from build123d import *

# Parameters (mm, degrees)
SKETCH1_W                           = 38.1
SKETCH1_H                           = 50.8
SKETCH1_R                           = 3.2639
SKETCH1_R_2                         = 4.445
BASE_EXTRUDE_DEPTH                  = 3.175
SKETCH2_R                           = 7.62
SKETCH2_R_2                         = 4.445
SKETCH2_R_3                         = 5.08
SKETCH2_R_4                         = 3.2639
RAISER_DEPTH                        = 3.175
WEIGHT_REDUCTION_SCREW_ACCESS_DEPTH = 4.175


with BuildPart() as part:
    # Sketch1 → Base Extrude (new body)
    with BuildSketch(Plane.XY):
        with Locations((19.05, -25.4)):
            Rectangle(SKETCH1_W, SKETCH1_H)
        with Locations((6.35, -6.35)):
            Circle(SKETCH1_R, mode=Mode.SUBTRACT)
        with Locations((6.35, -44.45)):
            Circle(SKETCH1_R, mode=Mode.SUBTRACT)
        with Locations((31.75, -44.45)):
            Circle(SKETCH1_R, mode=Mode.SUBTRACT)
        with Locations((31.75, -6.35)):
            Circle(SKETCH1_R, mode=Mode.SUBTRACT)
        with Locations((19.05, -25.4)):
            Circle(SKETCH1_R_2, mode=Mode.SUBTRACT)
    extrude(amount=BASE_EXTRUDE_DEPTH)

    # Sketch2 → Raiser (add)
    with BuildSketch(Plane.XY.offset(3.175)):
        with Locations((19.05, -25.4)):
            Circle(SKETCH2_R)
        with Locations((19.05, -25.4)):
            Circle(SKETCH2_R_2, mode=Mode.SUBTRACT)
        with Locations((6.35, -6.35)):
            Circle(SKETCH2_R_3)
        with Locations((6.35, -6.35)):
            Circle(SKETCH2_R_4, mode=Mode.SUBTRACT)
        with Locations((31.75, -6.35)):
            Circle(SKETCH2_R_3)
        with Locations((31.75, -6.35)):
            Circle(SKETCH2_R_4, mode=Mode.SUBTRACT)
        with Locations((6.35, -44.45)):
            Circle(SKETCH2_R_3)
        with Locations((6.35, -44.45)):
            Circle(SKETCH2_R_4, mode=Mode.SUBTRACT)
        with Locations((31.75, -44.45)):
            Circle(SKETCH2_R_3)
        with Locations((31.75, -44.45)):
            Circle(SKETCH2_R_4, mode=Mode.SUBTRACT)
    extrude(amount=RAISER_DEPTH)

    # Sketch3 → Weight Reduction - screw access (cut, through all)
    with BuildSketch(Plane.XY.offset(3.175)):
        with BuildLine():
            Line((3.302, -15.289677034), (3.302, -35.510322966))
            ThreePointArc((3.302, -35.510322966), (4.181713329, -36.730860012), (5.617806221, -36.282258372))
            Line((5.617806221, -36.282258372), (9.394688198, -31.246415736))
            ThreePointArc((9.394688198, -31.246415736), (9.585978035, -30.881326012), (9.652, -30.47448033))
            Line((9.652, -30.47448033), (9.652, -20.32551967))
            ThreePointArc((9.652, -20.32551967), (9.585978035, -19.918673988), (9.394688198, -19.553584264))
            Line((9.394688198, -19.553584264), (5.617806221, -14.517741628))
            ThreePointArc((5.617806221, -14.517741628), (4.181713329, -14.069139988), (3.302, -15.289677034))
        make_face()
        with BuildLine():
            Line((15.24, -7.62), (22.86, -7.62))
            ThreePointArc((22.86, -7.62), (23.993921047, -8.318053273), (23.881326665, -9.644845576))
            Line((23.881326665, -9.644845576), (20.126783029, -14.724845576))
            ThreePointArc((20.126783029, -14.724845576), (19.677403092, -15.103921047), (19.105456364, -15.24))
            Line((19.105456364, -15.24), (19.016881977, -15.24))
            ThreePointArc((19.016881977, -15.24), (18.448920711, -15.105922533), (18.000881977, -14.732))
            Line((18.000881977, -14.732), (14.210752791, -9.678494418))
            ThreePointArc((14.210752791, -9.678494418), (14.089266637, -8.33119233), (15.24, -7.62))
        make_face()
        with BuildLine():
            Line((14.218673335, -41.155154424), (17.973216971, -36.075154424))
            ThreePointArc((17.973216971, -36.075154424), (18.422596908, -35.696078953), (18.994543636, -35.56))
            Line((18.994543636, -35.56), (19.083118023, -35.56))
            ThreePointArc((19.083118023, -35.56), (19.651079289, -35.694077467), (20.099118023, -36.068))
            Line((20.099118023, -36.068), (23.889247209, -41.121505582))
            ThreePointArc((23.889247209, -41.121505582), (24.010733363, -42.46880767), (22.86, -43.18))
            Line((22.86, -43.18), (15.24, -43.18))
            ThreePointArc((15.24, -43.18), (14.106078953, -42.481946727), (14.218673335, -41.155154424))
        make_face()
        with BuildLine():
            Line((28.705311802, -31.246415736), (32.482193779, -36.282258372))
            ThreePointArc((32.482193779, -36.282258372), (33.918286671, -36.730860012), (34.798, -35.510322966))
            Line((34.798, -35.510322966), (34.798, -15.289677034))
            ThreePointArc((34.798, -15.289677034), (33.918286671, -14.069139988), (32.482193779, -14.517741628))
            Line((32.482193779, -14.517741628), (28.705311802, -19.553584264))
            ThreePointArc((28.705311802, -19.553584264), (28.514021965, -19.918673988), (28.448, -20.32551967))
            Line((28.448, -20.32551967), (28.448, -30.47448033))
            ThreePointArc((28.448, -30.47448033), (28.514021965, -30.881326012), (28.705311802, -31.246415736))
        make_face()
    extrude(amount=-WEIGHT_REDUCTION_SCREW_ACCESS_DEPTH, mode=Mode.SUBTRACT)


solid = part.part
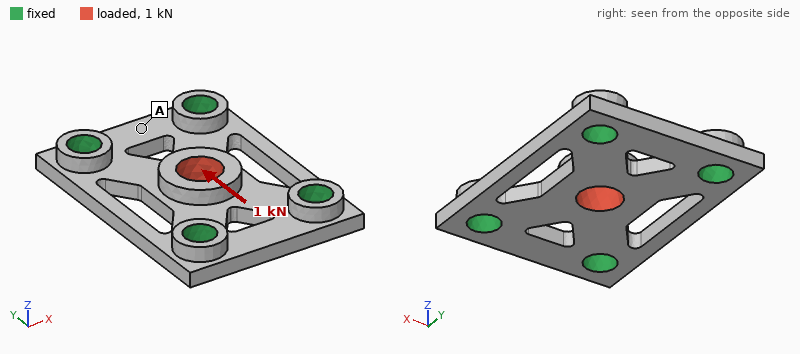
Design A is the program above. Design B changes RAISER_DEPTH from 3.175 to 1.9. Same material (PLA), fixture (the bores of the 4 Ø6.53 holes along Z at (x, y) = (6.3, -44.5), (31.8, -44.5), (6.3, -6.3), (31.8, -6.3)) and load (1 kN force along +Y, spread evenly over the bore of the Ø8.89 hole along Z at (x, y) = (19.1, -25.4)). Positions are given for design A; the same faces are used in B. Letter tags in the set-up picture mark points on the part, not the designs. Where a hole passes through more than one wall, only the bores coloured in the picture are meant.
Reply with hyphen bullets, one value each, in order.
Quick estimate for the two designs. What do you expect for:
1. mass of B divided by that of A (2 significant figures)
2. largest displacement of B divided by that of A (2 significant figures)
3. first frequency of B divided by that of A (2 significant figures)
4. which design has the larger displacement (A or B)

- 0.93
- 0.71
- 1.0
- A
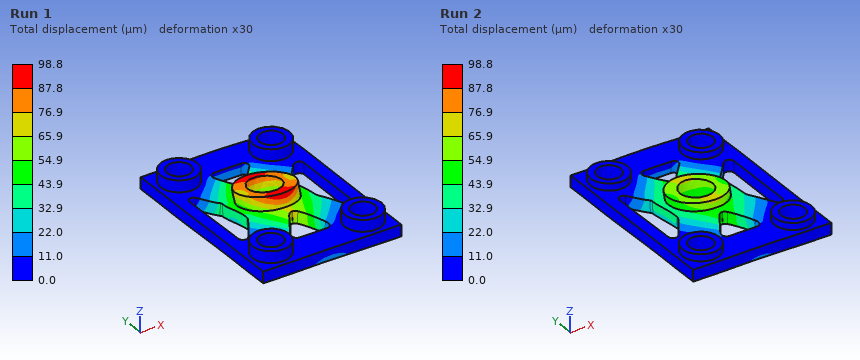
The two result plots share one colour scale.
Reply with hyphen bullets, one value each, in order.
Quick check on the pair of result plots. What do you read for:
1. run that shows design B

- Run 2
